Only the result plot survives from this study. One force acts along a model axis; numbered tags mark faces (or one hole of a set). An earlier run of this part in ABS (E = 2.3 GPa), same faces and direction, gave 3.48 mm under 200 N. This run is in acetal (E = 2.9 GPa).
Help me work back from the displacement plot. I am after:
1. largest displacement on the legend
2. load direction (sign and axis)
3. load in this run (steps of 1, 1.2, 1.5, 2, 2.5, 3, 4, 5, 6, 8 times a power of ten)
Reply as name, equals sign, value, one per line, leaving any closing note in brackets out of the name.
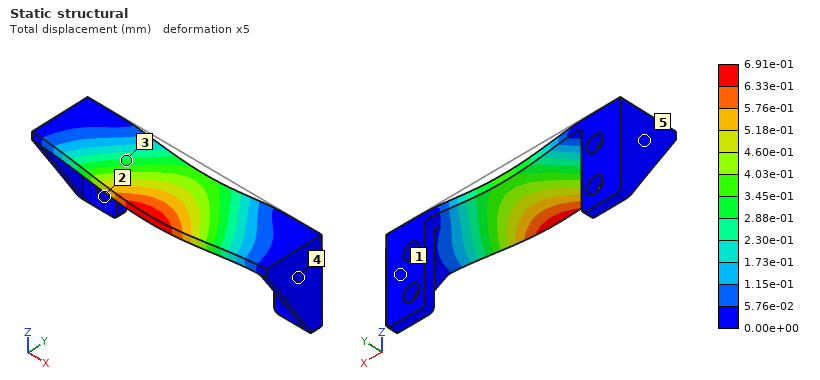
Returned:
largest displacement on the legend = 6.91e-01 mm
load direction = -Z
load in this run = 50 N
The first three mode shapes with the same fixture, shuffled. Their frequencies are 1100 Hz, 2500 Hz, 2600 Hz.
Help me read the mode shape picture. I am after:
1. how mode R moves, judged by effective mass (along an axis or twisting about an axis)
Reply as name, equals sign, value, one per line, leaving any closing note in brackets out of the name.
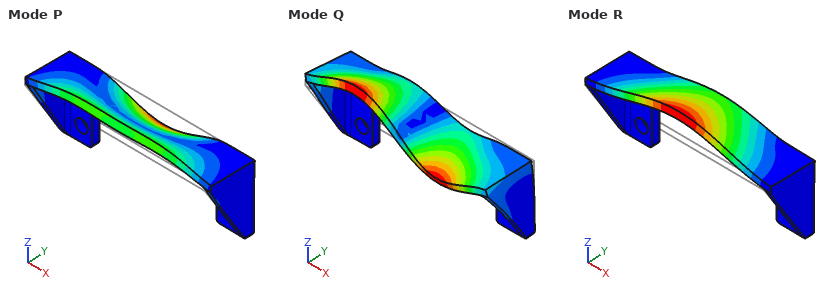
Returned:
how mode R moves, judged by effective mass = along Z
